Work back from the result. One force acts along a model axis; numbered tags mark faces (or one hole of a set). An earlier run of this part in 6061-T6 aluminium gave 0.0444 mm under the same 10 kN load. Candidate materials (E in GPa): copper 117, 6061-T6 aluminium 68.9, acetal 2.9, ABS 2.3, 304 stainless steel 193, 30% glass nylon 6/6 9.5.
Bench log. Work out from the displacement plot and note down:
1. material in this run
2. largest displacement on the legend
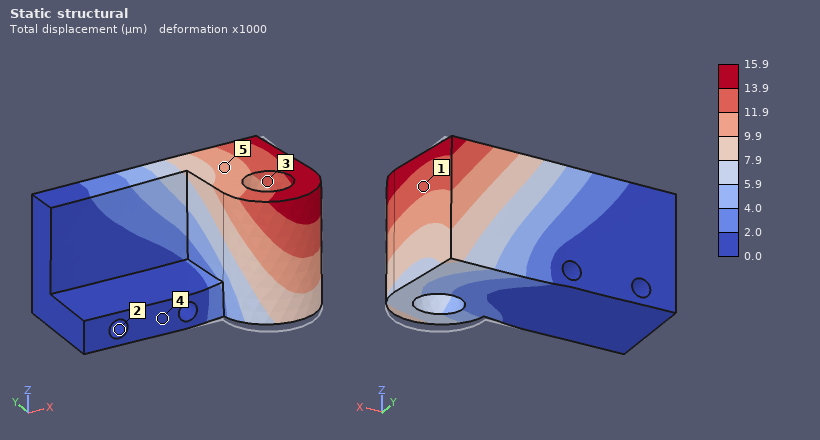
304 stainless steel
15.9 µm
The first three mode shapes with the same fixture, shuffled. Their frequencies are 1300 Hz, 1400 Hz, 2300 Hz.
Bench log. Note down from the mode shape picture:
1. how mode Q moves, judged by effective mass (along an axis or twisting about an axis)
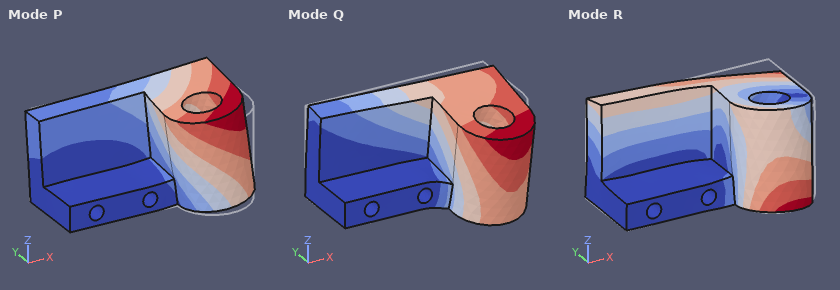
along Y
